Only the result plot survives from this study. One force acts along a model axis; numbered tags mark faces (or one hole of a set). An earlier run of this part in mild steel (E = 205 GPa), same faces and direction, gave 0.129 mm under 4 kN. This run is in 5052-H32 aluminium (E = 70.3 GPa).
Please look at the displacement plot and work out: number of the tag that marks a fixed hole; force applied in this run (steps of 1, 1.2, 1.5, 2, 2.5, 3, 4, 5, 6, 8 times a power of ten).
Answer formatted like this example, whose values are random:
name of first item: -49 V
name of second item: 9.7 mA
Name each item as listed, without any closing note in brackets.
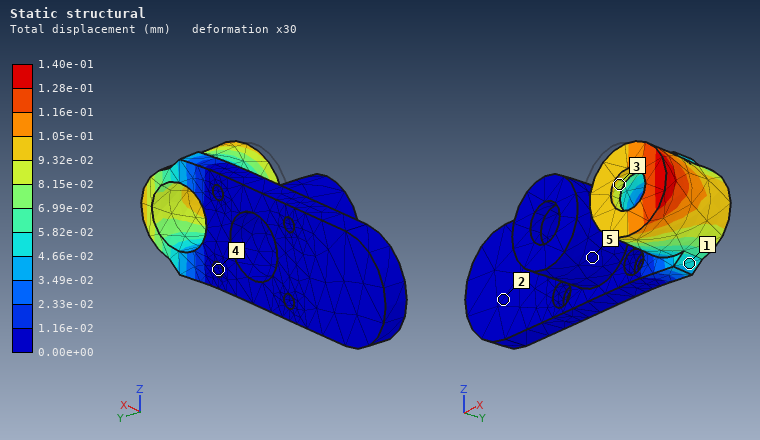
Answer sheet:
number of the tag that marks a fixed hole: 4
force applied in this run: 1.5 kN
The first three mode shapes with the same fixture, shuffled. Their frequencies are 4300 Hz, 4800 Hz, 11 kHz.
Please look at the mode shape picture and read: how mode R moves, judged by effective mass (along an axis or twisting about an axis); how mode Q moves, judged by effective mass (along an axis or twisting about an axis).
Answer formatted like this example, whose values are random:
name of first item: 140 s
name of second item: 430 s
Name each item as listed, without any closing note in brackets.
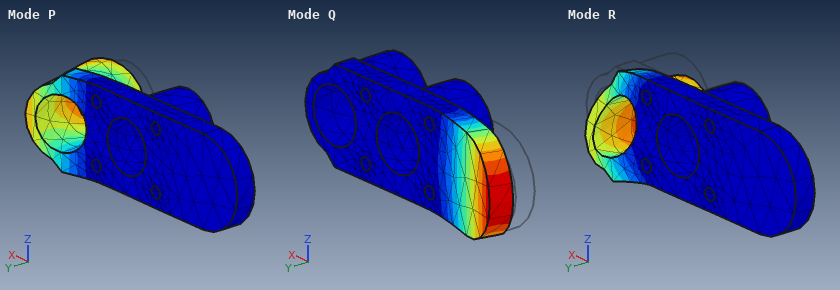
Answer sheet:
how mode R moves, judged by effective mass: along Z
how mode Q moves, judged by effective mass: along Y
